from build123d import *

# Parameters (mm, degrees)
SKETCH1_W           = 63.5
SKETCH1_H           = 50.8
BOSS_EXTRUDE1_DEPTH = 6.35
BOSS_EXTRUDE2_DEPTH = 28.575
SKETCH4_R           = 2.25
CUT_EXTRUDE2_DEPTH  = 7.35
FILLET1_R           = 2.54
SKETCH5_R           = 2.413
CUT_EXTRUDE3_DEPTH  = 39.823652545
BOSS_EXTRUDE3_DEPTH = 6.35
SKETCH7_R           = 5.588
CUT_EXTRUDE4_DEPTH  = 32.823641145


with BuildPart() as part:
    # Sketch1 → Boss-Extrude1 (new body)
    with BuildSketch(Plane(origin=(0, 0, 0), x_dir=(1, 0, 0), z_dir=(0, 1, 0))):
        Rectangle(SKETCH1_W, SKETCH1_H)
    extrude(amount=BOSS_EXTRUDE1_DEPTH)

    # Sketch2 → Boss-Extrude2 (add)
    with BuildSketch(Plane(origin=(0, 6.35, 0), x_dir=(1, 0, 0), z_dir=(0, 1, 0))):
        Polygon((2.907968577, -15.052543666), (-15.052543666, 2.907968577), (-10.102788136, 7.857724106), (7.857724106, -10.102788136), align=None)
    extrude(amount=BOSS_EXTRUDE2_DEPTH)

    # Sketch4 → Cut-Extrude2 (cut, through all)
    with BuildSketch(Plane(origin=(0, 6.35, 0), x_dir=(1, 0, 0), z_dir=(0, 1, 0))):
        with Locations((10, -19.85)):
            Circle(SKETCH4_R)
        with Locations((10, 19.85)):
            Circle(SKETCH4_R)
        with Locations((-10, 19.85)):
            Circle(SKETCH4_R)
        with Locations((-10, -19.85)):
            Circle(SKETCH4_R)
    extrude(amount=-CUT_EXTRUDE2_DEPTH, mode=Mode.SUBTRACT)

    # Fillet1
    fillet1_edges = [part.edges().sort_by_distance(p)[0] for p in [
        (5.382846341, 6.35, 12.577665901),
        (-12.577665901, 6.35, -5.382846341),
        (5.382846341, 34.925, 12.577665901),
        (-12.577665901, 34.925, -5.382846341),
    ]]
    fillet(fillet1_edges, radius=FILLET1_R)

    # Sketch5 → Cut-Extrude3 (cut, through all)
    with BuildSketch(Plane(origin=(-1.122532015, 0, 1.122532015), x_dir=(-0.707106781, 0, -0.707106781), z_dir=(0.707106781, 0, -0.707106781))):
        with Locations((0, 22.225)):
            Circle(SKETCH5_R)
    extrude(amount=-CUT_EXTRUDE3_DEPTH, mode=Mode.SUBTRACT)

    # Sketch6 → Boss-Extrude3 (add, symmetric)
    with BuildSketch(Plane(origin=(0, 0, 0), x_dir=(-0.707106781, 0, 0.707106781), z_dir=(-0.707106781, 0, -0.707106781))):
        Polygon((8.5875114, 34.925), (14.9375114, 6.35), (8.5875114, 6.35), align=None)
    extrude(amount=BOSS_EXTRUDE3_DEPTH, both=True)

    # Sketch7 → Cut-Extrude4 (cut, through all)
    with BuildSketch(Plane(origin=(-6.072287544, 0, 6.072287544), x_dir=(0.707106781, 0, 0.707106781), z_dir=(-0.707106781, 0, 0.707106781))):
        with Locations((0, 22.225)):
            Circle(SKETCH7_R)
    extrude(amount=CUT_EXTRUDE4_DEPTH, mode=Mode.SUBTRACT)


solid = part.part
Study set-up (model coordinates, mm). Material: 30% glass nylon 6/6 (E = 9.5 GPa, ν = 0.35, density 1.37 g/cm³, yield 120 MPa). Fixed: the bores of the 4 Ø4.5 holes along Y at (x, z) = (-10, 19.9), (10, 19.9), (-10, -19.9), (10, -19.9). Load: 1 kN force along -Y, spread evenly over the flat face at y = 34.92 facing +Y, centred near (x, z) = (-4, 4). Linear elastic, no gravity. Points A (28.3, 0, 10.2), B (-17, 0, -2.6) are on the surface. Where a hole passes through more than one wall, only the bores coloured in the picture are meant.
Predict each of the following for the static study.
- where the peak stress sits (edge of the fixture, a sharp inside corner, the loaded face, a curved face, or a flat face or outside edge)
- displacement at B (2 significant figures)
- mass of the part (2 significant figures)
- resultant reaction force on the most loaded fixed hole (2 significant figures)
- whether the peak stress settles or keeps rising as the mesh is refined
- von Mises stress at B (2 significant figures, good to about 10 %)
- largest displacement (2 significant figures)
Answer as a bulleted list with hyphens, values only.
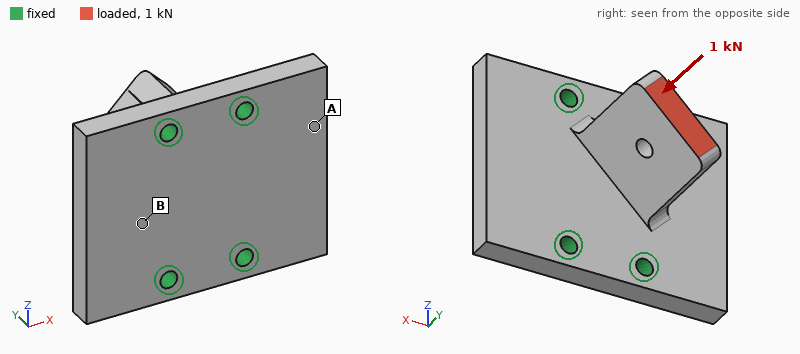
- edge of the fixture
- 32 µm
- 35 g
- 330 N
- keeps rising
- 7.1 MPa
- 76 µm
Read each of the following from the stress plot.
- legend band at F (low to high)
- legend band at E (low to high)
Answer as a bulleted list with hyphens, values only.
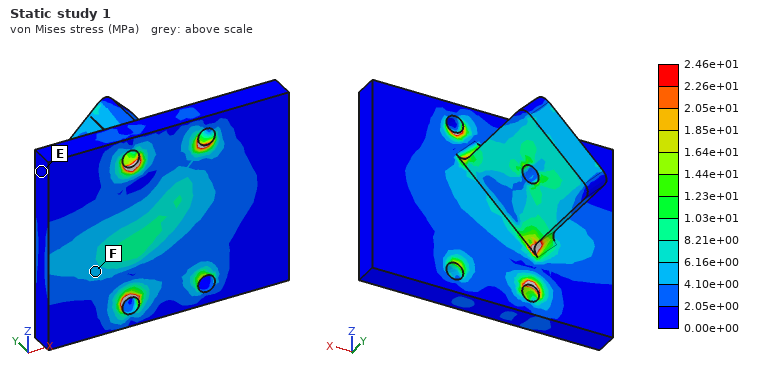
- 4.10e+00 to 6.16e+00 MPa
- 0.00e+00 to 2.05e+00 MPa
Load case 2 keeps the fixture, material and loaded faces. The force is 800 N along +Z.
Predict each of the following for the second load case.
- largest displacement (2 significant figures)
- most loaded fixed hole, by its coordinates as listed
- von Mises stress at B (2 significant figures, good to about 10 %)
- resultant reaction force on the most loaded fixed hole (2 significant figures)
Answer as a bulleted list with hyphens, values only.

- 0.50 mm
- (-10, 19.9)
- 14 MPa
- 740 N
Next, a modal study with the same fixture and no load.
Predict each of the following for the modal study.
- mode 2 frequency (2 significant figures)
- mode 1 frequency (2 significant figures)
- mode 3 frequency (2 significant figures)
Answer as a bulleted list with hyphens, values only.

- 4500 Hz
- 3800 Hz
- 4600 Hz
